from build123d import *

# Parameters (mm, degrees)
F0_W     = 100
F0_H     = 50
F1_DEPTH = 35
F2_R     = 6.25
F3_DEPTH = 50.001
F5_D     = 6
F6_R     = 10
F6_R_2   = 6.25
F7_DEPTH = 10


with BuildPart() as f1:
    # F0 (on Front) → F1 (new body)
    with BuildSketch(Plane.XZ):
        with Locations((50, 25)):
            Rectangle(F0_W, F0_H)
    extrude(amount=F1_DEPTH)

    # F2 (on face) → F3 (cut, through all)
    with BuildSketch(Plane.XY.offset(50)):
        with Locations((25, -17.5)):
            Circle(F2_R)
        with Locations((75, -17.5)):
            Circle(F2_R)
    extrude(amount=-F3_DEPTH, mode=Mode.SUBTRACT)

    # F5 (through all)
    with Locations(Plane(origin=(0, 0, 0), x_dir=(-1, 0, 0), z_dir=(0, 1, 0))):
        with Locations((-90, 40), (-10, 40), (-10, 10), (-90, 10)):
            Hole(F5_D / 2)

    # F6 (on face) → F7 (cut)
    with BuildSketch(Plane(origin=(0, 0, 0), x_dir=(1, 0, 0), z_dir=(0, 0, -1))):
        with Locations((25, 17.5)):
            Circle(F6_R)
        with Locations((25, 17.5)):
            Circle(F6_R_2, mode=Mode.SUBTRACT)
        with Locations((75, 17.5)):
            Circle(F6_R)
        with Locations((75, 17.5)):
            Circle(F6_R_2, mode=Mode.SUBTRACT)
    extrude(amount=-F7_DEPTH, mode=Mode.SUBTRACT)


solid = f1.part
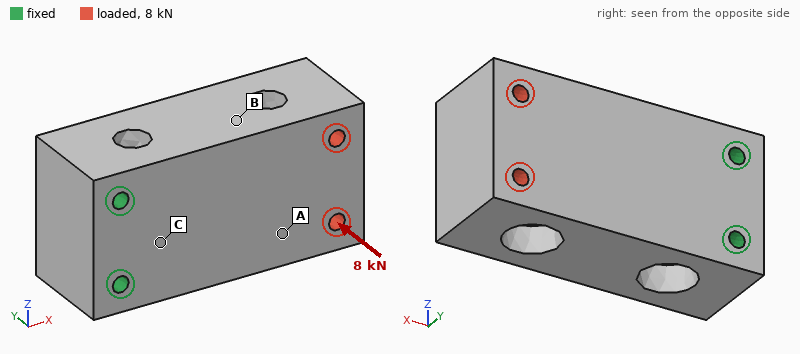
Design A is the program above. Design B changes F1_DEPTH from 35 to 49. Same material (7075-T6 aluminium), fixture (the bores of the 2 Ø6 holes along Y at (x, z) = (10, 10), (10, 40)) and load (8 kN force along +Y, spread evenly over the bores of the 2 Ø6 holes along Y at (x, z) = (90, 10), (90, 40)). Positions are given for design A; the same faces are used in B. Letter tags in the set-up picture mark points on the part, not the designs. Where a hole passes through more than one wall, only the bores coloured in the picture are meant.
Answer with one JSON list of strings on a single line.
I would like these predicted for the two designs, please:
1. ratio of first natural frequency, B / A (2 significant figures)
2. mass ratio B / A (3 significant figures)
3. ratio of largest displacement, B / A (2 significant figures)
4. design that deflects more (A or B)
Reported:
["1.2", "1.44", "0.42", "A"]
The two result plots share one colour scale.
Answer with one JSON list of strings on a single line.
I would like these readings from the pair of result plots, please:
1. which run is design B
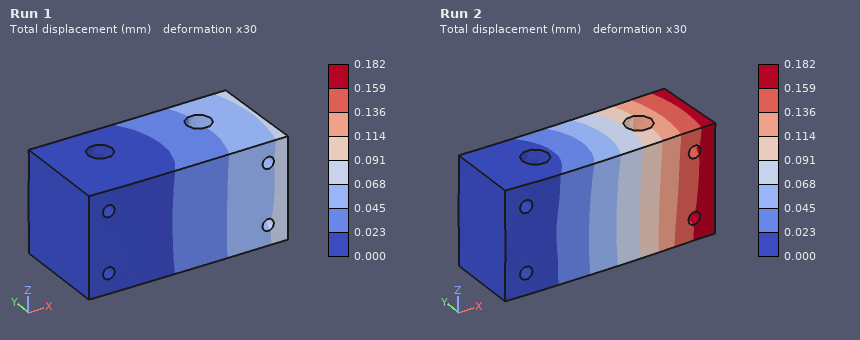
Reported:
["Run 1"]
